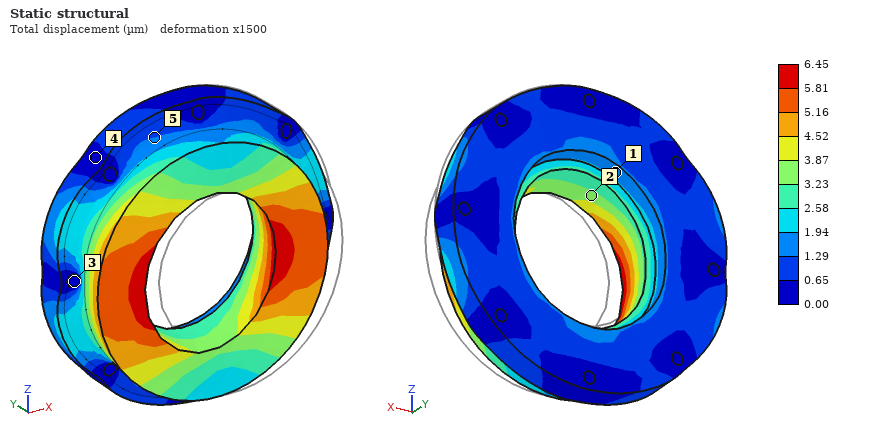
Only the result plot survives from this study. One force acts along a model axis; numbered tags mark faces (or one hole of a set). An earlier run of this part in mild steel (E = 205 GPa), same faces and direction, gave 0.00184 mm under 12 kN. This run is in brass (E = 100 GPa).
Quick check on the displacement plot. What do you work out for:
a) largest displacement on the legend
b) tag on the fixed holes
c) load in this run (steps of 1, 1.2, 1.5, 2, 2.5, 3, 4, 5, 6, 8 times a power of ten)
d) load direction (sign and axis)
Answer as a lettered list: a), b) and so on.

a) 6.45 µm
b) 3
c) 20 kN
d) -X
